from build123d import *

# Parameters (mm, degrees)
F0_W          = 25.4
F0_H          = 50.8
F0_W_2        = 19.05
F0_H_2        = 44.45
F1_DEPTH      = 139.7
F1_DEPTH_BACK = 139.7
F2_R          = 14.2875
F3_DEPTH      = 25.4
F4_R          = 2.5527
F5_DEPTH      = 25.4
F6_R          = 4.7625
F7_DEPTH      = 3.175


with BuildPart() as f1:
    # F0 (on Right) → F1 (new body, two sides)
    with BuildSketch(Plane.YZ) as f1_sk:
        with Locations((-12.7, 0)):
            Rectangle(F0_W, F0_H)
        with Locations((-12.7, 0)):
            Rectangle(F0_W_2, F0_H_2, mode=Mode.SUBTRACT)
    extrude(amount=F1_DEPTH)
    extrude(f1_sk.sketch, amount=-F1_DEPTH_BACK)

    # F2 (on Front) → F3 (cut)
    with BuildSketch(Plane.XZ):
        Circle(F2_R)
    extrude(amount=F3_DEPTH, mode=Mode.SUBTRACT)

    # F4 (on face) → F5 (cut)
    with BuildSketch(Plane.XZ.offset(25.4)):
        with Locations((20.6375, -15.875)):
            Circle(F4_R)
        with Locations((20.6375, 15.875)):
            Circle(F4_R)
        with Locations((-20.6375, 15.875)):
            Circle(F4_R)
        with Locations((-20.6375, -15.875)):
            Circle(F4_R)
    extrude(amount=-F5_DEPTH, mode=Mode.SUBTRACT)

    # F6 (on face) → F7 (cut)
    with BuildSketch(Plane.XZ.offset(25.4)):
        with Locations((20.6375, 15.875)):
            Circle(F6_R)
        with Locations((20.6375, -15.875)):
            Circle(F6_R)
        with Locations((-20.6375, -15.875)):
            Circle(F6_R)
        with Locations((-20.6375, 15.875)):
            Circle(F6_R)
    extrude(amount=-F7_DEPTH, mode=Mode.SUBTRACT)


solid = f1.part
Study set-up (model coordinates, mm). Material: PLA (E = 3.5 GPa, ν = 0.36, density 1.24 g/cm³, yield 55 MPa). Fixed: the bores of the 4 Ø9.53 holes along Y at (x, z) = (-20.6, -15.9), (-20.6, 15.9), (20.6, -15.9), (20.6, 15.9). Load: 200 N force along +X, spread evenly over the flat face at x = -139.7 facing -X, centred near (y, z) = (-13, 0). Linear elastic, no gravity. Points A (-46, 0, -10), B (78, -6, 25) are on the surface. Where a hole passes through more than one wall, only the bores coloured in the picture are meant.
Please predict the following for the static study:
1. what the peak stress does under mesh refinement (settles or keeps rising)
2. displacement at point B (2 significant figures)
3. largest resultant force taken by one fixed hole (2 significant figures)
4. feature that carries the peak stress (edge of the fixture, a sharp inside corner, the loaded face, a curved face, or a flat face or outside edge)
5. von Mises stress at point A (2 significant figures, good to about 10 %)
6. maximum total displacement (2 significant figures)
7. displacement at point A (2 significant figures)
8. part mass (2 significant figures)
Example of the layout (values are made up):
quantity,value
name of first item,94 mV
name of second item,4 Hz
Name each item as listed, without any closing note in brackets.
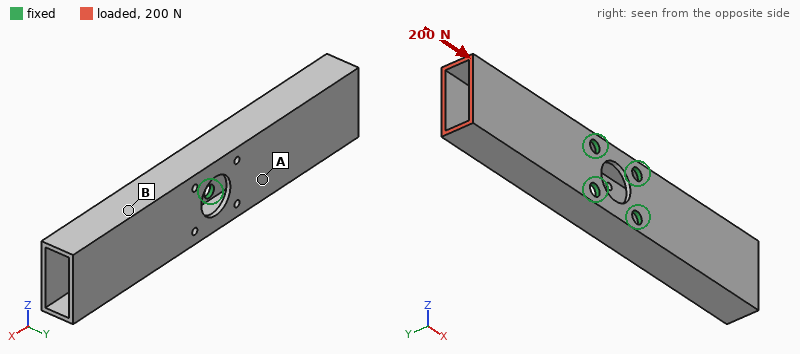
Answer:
quantity,value
what the peak stress does under mesh refinement,keeps rising
displacement at point B,26 µm
largest resultant force taken by one fixed hole,74 N
feature that carries the peak stress,edge of the fixture
von Mises stress at point A,0.42 MPa
maximum total displacement,88 µm
displacement at point A,28 µm
part mass,150 g
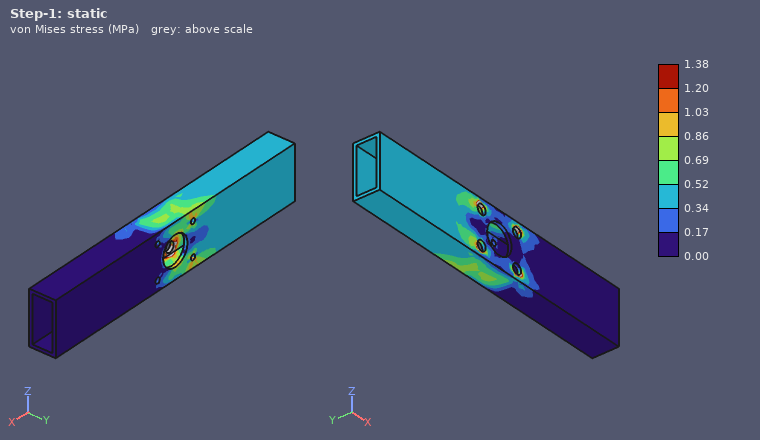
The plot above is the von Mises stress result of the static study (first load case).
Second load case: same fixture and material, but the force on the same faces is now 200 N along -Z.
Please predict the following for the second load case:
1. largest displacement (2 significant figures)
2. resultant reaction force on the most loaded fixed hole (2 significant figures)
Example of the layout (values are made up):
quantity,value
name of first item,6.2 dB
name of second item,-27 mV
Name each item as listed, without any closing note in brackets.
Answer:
quantity,value
largest displacement,0.51 mm
resultant reaction force on the most loaded fixed hole,480 N
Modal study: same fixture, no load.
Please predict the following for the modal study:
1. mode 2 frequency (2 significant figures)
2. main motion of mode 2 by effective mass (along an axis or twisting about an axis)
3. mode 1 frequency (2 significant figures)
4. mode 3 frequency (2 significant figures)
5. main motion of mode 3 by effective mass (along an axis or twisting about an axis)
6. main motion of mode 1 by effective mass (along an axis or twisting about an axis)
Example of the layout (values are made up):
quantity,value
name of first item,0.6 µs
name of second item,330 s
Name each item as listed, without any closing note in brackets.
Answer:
quantity,value
mode 2 frequency,450 Hz
main motion of mode 2 by effective mass,along Y
mode 1 frequency,320 Hz
mode 3 frequency,570 Hz
main motion of mode 3 by effective mass,along Z
main motion of mode 1 by effective mass,twisting about Z
